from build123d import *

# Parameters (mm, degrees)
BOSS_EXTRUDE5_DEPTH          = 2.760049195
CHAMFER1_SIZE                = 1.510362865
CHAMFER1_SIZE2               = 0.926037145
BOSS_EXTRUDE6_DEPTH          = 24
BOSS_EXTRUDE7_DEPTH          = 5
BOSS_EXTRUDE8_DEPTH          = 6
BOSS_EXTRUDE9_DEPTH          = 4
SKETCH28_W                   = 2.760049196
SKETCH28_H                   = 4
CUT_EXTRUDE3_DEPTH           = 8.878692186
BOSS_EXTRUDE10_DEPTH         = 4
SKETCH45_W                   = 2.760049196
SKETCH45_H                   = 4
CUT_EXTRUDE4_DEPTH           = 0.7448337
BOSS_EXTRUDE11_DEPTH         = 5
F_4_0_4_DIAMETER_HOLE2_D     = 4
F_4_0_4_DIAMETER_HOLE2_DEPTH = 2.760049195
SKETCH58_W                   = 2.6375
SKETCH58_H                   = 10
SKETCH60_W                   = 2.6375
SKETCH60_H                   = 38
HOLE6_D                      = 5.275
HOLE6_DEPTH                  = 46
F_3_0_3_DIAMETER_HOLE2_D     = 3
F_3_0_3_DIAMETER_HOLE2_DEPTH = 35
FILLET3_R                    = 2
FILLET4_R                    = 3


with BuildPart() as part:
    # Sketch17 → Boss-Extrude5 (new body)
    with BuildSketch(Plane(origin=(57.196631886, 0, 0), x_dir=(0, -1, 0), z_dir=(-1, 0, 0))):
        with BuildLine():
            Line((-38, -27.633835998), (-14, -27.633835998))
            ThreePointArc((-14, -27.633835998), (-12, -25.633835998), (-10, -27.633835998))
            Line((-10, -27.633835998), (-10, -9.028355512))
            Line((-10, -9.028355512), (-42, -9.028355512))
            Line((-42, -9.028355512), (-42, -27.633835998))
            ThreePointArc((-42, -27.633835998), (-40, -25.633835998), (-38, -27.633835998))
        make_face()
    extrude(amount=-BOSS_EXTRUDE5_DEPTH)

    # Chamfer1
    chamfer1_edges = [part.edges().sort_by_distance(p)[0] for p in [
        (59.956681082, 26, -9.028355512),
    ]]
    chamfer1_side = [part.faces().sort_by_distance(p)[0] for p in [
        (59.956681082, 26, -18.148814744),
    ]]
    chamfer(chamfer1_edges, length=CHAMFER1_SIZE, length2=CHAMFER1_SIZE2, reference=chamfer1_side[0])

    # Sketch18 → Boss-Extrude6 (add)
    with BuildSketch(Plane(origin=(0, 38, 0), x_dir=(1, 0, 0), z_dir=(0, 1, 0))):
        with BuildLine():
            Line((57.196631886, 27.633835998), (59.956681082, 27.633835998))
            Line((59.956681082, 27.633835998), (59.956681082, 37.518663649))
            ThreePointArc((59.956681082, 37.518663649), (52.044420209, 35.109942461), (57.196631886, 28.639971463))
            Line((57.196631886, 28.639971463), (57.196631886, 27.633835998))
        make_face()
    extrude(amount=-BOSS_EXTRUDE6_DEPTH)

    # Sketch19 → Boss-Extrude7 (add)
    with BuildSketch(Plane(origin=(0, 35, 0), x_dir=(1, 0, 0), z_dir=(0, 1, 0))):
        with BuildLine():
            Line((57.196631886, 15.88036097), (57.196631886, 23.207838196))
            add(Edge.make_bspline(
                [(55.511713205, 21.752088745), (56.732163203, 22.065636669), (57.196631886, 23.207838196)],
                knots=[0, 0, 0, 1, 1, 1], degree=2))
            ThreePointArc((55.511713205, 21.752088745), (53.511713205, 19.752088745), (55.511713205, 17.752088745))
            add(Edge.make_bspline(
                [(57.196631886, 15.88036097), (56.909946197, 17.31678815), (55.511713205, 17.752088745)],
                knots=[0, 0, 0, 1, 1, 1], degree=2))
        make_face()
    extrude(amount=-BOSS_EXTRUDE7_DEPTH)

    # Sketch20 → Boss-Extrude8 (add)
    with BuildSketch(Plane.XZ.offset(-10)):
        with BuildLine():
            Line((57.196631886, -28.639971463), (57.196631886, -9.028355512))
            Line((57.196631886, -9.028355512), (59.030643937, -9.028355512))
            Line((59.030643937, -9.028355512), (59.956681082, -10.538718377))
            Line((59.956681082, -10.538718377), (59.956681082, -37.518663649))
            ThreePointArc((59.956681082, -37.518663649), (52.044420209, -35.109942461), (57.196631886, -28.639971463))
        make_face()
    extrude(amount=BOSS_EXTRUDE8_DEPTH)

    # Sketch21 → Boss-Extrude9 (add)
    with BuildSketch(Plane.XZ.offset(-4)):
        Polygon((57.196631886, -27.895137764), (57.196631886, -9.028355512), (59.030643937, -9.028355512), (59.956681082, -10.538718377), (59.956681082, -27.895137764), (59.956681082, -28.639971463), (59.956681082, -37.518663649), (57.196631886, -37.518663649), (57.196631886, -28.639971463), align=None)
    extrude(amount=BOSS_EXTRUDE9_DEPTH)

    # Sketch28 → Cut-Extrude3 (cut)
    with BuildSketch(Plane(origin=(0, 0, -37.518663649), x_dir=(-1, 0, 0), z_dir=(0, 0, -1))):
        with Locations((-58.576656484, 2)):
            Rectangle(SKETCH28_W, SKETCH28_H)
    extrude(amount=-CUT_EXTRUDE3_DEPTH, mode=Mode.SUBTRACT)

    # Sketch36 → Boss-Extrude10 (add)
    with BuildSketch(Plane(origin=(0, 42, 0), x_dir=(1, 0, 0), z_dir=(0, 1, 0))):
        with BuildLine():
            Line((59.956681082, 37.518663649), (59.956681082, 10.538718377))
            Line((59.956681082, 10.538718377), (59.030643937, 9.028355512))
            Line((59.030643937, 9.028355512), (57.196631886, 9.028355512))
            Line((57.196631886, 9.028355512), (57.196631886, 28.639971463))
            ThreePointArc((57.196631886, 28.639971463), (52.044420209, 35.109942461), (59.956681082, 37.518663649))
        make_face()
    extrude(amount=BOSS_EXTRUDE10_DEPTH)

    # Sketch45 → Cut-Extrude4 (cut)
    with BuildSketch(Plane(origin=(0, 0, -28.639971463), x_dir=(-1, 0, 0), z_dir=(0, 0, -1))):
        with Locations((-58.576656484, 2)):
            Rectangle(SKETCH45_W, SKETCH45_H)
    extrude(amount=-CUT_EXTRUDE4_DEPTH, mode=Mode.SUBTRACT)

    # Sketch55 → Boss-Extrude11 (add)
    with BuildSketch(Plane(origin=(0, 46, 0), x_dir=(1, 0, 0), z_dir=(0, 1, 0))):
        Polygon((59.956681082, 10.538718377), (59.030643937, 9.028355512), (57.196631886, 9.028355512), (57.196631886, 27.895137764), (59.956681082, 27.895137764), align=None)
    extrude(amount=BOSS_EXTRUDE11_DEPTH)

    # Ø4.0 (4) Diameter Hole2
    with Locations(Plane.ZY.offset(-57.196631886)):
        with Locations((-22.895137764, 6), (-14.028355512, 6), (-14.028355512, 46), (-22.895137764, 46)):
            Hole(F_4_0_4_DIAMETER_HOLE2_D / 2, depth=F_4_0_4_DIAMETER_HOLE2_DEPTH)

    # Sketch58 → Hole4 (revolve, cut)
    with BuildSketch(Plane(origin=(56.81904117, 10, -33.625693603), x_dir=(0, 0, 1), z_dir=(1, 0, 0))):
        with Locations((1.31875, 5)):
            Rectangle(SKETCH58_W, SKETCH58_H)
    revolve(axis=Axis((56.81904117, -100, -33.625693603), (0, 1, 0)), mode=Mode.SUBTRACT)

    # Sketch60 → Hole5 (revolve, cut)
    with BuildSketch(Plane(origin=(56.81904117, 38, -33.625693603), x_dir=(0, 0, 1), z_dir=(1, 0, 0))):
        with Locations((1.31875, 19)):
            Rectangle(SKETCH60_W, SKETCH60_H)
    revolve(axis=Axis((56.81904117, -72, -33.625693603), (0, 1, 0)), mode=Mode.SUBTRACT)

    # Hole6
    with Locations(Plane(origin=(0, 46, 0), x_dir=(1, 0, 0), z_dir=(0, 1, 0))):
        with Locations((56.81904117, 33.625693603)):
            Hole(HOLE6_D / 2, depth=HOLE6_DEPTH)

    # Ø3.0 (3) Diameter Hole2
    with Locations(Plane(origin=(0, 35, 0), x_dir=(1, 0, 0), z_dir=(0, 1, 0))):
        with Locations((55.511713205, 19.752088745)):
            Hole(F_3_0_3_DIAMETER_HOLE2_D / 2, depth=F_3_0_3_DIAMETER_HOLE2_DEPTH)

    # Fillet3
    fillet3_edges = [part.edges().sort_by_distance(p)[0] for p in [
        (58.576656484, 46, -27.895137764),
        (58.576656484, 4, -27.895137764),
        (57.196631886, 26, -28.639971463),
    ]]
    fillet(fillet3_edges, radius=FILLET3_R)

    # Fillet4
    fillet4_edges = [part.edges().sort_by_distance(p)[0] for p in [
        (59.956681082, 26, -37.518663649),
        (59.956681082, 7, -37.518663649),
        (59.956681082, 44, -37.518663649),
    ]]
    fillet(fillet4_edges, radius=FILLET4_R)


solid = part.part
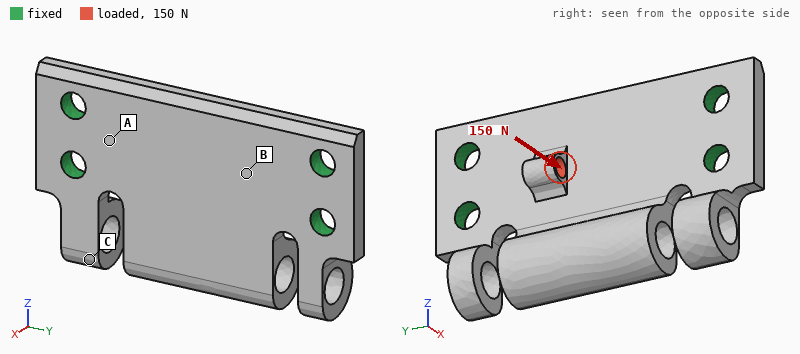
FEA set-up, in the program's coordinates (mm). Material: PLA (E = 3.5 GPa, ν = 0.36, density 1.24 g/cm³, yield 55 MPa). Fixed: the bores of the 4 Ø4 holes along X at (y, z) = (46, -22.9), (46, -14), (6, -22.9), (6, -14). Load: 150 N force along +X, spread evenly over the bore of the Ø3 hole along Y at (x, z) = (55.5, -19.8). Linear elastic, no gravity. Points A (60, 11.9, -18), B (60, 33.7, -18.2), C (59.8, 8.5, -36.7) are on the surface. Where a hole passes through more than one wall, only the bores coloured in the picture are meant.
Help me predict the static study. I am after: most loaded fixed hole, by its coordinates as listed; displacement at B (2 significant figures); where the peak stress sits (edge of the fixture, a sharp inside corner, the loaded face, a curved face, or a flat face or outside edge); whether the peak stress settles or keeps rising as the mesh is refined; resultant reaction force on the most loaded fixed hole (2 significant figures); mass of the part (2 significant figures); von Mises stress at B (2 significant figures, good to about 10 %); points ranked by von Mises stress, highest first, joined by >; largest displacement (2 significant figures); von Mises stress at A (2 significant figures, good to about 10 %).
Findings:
(46, -22.9)
0.18 mm
edge of the fixture
keeps rising
67 N
5.2 g
14 MPa
B > A > C
0.23 mm
6.2 MPa
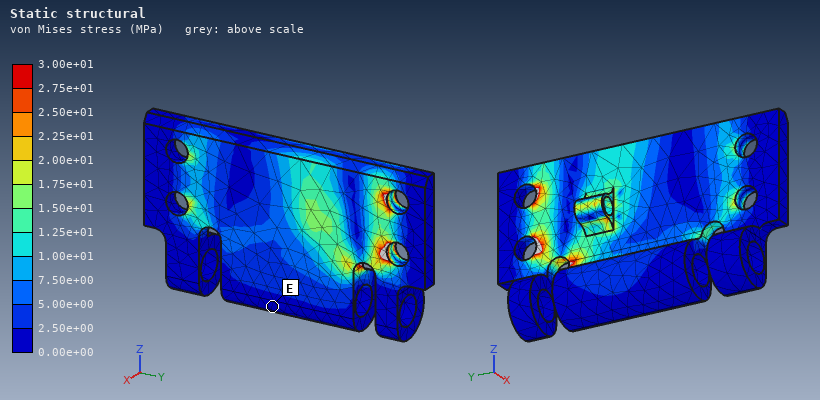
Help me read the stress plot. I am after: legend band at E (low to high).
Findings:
0.00e+00 to 2.50e+00 MPa
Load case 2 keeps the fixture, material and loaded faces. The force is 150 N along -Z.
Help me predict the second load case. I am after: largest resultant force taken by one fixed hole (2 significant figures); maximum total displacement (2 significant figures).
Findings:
81 N
0.21 mm
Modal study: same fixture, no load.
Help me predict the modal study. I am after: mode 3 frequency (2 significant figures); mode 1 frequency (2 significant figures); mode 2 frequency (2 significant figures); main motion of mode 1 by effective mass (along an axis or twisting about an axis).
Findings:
2900 Hz
1400 Hz
2800 Hz
along X
